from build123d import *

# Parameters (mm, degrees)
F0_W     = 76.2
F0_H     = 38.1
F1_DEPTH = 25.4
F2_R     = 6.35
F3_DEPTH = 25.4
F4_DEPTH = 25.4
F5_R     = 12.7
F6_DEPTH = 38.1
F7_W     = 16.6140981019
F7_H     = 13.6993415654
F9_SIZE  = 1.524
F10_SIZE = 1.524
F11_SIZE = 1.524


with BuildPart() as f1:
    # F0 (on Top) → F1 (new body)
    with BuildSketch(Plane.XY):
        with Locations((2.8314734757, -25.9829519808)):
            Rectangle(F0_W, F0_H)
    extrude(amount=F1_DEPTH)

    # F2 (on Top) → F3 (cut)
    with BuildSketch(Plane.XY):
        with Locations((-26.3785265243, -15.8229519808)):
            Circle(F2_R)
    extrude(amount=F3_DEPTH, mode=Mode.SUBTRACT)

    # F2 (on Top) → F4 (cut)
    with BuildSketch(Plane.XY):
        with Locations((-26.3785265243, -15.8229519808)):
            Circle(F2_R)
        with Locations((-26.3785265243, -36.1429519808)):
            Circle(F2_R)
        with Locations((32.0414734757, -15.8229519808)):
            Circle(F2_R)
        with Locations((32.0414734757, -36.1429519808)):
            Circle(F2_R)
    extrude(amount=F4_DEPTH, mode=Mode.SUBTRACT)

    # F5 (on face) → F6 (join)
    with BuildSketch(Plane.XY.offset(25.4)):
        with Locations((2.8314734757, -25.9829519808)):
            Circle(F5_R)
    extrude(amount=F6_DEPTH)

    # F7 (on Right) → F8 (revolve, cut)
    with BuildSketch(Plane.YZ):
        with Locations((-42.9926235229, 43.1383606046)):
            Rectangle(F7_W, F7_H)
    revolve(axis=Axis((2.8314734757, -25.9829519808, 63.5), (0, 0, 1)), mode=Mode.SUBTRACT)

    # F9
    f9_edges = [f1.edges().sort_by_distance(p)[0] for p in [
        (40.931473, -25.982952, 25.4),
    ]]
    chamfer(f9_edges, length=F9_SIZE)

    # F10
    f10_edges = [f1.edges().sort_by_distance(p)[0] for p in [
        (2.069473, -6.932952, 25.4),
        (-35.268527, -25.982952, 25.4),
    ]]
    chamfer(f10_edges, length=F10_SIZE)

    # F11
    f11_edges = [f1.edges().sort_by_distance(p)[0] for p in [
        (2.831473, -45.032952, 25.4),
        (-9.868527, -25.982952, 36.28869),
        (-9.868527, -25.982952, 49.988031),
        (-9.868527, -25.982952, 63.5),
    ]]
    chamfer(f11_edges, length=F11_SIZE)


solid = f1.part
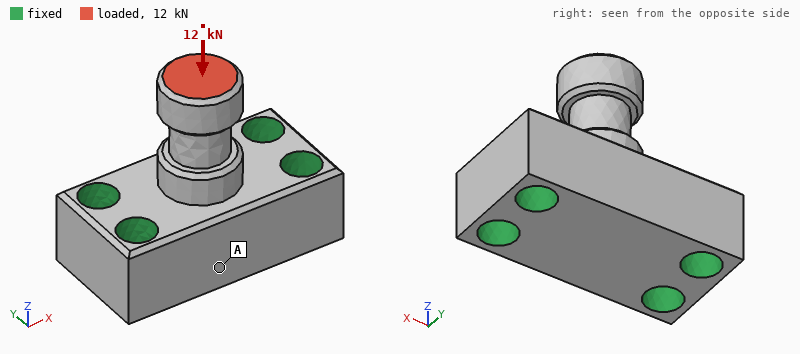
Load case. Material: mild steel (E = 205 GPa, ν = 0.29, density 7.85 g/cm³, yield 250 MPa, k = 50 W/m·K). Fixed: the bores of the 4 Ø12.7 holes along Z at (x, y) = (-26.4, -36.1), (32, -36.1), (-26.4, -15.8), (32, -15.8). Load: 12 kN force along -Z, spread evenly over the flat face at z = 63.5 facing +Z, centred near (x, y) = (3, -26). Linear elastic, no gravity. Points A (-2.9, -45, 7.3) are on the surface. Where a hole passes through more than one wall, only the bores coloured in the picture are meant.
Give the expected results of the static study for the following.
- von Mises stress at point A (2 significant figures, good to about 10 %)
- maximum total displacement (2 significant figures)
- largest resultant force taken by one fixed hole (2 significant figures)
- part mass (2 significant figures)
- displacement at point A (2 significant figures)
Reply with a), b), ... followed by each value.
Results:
a) 6.4 MPa
b) 9.1 µm
c) 3.1 kN
d) 600 g
e) 1.6 µm
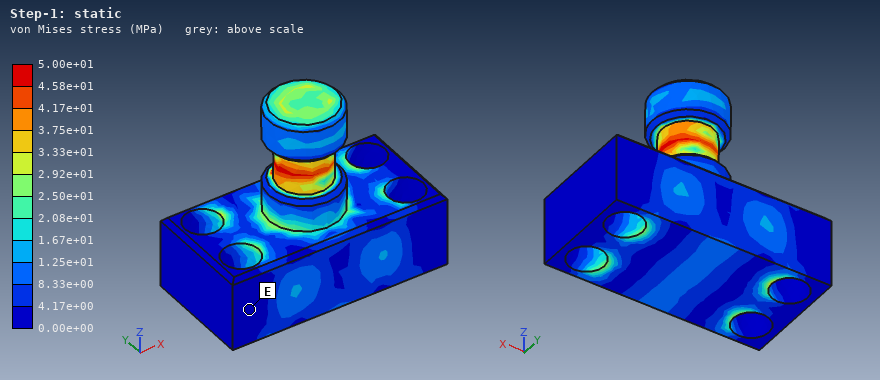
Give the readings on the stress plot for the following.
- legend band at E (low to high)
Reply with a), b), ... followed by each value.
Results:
a) 0.00e+00 to 4.17e+00 MPa
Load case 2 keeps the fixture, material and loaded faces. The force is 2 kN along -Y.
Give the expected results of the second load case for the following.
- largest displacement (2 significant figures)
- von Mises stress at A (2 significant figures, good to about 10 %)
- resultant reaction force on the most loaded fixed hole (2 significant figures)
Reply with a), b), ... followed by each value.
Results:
a) 32 µm
b) 6.5 MPa
c) 1.6 kN
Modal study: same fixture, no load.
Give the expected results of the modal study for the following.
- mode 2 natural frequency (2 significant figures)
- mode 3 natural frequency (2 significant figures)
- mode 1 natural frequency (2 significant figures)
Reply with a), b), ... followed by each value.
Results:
a) 7200 Hz
b) 15 kHz
c) 6600 Hz
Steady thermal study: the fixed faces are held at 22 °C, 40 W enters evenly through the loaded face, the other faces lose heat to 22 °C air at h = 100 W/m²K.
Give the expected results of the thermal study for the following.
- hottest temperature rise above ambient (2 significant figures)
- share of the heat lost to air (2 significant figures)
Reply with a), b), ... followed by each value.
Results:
a) 79 K
b) 36 %
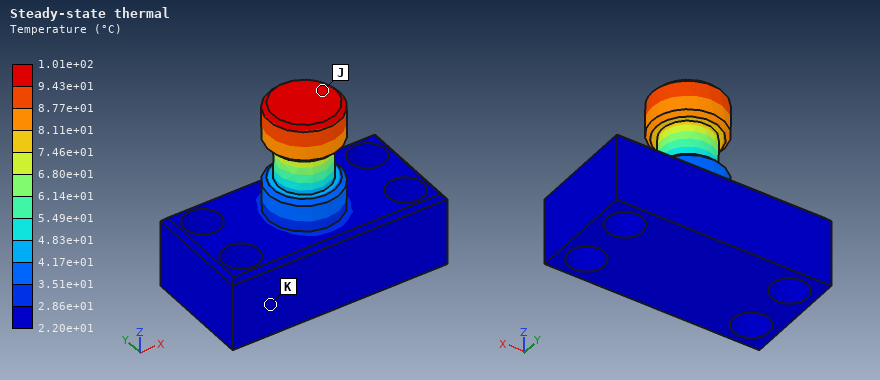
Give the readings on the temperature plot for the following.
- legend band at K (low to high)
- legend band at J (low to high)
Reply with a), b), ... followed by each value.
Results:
a) 2.20e+01 to 2.86e+01 °C
b) 9.43e+01 to 1.01e+02 °C
